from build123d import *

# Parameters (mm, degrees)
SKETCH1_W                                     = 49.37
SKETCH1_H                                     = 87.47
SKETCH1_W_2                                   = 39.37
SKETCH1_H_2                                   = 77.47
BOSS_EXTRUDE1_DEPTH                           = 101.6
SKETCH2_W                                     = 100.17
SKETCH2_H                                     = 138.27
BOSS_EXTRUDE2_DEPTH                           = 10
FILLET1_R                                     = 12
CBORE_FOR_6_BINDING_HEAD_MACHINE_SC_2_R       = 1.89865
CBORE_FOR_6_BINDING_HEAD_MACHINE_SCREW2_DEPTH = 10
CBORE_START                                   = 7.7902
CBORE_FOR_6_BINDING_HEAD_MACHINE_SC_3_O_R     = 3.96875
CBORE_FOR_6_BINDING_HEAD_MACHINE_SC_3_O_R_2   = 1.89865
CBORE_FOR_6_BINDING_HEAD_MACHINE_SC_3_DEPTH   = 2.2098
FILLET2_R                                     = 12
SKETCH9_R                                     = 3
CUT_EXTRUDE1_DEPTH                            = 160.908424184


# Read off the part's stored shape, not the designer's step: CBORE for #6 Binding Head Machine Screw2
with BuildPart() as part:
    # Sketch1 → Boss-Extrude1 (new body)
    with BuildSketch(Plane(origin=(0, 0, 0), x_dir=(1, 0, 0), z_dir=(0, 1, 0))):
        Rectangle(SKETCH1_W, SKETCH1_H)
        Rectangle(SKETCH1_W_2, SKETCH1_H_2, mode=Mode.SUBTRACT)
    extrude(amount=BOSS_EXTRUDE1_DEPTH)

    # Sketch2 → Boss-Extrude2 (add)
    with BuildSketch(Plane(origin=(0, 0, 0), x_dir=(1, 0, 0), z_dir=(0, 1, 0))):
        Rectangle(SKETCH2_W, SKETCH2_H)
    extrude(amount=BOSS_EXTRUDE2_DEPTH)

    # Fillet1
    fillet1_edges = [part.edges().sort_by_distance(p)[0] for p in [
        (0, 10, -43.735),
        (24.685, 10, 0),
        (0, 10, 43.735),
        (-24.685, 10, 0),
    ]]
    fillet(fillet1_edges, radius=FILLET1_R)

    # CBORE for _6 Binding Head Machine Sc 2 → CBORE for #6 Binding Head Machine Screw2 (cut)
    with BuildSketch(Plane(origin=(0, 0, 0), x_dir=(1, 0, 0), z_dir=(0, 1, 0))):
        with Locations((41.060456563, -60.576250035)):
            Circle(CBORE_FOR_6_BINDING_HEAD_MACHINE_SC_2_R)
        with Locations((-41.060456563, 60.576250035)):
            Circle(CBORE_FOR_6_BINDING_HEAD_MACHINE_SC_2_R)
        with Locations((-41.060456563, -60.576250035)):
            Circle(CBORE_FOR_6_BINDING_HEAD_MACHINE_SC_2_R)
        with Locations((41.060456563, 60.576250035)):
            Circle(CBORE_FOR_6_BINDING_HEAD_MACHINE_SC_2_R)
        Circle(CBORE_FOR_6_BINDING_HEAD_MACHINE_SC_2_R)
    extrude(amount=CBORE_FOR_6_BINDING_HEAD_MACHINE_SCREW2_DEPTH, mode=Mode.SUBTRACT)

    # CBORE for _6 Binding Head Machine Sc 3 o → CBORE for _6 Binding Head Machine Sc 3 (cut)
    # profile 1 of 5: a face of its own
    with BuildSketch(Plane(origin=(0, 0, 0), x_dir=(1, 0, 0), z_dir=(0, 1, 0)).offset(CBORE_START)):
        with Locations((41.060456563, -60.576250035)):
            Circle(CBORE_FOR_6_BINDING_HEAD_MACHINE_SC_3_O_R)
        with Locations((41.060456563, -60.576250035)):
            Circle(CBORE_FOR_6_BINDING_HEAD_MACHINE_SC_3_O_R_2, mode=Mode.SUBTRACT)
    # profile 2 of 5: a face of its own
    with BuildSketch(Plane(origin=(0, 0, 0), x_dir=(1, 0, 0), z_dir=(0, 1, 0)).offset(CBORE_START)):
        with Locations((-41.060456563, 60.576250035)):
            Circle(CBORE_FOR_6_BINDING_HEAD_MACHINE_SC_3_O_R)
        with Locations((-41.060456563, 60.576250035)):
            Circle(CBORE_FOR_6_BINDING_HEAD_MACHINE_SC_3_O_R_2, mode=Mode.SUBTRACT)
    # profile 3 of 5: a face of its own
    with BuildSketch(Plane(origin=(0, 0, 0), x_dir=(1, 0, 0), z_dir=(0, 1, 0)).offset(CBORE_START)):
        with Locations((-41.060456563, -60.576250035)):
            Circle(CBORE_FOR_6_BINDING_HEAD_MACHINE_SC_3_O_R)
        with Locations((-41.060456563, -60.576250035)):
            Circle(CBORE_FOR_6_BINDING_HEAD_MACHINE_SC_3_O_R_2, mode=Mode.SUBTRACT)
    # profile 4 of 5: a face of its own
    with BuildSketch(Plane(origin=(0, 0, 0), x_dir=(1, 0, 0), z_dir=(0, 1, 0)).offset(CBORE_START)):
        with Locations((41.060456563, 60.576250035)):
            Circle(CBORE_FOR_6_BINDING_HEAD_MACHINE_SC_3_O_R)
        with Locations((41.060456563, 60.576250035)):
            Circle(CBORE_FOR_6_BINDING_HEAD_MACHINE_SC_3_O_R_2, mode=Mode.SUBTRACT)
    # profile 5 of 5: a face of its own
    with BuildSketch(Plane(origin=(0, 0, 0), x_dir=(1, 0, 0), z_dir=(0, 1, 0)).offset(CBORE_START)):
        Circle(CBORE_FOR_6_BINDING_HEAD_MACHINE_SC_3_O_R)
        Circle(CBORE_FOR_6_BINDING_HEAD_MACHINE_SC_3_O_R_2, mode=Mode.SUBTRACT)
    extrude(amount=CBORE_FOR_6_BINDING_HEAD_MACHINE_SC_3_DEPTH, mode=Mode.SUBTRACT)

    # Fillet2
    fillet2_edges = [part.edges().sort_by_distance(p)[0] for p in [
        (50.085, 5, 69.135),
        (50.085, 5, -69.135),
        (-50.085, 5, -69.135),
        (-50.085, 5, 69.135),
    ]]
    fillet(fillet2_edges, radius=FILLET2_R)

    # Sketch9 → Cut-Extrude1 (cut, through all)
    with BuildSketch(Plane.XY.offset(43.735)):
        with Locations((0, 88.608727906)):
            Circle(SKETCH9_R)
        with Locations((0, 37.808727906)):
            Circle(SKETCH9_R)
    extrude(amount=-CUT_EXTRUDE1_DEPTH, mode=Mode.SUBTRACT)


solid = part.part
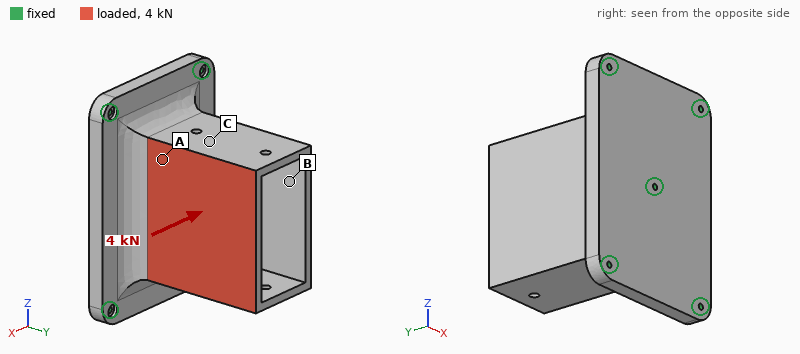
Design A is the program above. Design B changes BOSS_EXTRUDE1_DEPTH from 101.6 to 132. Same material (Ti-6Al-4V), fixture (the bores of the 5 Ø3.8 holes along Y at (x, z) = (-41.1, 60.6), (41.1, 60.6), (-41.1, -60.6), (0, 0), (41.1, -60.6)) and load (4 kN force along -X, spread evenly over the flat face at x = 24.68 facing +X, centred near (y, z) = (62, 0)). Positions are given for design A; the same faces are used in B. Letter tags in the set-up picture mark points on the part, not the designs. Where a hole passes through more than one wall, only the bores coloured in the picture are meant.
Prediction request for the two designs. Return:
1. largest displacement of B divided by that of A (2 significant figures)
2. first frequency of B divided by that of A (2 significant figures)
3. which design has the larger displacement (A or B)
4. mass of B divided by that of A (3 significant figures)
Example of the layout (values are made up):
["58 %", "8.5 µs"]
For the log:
["1.1", "0.71", "B", "1.15"]
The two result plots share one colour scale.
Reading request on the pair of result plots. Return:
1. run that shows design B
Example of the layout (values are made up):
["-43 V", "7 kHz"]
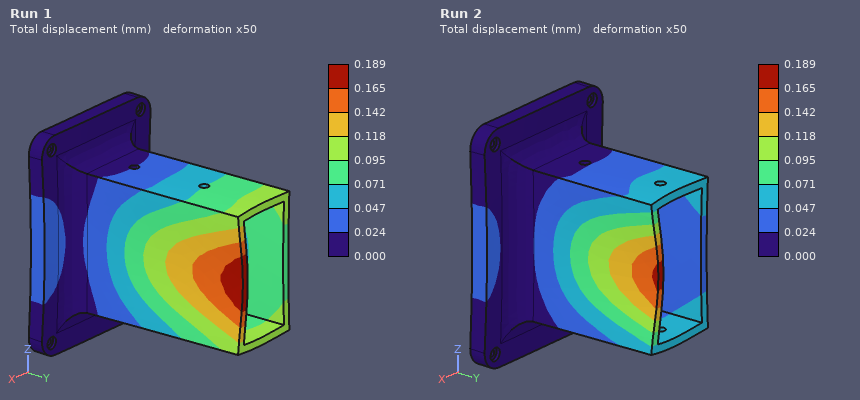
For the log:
["Run 1"]
